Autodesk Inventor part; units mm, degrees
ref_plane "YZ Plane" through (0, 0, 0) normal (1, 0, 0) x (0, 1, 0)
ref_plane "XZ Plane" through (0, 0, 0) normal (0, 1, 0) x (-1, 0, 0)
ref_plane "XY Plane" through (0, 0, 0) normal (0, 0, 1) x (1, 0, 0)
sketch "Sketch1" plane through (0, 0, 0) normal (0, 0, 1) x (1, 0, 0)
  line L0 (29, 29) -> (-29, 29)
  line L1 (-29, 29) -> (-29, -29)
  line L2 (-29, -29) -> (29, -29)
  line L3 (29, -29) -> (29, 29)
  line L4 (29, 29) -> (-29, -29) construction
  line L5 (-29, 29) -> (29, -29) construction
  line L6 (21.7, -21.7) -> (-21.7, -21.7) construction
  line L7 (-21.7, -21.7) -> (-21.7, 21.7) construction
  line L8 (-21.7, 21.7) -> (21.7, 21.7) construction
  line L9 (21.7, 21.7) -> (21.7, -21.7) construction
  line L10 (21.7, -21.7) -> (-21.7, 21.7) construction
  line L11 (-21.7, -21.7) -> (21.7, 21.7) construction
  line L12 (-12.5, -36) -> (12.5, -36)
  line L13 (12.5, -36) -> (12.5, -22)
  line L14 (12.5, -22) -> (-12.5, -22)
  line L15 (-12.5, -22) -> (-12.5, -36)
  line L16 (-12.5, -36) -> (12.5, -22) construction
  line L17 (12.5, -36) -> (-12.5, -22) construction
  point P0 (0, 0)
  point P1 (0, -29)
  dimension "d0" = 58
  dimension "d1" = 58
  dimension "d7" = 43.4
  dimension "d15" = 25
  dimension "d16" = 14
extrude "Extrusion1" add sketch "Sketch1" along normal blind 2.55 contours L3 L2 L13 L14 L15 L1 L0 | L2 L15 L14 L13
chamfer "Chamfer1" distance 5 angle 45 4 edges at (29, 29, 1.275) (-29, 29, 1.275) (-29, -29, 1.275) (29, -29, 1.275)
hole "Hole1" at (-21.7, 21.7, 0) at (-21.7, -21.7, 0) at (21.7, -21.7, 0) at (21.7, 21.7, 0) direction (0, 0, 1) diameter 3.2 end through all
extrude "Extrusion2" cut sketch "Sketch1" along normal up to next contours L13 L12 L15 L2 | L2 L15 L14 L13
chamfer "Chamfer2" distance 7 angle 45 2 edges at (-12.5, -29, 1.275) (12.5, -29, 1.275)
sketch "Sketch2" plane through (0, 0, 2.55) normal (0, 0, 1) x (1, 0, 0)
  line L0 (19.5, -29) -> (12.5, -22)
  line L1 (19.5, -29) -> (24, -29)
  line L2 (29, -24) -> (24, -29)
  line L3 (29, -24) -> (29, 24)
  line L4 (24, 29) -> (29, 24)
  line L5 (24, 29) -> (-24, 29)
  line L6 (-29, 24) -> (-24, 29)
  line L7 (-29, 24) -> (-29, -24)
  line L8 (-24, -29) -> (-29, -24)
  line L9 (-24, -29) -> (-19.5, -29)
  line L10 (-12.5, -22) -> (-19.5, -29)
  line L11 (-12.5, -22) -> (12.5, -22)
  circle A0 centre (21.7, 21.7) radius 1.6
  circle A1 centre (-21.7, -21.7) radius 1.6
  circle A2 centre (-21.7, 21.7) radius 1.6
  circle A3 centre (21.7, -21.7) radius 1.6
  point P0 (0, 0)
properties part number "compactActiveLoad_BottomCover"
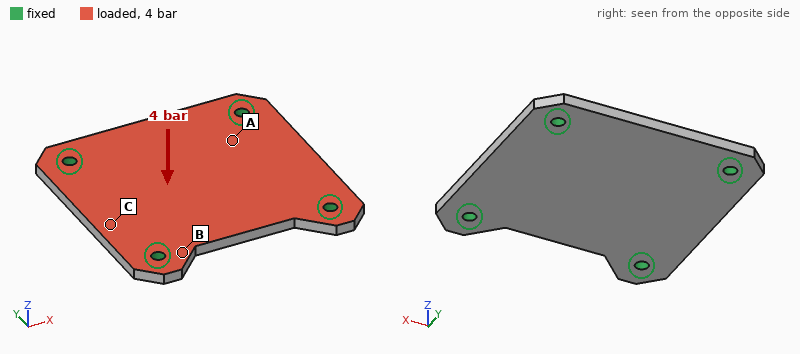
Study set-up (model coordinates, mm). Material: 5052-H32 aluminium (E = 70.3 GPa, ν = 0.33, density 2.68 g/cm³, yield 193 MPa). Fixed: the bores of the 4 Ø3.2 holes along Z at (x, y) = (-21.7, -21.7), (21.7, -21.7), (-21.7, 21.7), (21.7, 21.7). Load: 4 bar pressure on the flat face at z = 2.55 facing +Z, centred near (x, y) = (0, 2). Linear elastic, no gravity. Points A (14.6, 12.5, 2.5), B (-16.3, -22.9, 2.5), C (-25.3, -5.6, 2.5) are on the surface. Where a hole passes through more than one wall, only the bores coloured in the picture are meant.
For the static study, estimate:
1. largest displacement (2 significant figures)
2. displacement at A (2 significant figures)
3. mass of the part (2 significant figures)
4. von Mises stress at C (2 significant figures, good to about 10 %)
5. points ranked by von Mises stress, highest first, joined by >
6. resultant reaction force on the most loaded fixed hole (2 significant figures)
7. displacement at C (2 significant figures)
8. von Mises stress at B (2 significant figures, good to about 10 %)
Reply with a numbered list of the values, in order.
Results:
1. 90 µm
2. 43 µm
3. 21 g
4. 27 MPa
5. B > C > A
6. 330 N
7. 38 µm
8. 51 MPa
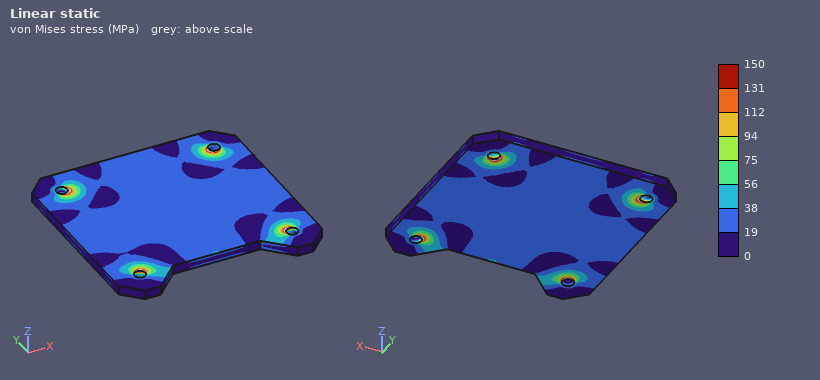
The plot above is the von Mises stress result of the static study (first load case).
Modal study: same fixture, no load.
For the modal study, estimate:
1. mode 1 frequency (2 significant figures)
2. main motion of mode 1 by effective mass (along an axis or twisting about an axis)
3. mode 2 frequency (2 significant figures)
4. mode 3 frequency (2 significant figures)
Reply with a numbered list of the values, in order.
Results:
1. 4900 Hz
2. along Z
3. 7700 Hz
4. 7800 Hz
